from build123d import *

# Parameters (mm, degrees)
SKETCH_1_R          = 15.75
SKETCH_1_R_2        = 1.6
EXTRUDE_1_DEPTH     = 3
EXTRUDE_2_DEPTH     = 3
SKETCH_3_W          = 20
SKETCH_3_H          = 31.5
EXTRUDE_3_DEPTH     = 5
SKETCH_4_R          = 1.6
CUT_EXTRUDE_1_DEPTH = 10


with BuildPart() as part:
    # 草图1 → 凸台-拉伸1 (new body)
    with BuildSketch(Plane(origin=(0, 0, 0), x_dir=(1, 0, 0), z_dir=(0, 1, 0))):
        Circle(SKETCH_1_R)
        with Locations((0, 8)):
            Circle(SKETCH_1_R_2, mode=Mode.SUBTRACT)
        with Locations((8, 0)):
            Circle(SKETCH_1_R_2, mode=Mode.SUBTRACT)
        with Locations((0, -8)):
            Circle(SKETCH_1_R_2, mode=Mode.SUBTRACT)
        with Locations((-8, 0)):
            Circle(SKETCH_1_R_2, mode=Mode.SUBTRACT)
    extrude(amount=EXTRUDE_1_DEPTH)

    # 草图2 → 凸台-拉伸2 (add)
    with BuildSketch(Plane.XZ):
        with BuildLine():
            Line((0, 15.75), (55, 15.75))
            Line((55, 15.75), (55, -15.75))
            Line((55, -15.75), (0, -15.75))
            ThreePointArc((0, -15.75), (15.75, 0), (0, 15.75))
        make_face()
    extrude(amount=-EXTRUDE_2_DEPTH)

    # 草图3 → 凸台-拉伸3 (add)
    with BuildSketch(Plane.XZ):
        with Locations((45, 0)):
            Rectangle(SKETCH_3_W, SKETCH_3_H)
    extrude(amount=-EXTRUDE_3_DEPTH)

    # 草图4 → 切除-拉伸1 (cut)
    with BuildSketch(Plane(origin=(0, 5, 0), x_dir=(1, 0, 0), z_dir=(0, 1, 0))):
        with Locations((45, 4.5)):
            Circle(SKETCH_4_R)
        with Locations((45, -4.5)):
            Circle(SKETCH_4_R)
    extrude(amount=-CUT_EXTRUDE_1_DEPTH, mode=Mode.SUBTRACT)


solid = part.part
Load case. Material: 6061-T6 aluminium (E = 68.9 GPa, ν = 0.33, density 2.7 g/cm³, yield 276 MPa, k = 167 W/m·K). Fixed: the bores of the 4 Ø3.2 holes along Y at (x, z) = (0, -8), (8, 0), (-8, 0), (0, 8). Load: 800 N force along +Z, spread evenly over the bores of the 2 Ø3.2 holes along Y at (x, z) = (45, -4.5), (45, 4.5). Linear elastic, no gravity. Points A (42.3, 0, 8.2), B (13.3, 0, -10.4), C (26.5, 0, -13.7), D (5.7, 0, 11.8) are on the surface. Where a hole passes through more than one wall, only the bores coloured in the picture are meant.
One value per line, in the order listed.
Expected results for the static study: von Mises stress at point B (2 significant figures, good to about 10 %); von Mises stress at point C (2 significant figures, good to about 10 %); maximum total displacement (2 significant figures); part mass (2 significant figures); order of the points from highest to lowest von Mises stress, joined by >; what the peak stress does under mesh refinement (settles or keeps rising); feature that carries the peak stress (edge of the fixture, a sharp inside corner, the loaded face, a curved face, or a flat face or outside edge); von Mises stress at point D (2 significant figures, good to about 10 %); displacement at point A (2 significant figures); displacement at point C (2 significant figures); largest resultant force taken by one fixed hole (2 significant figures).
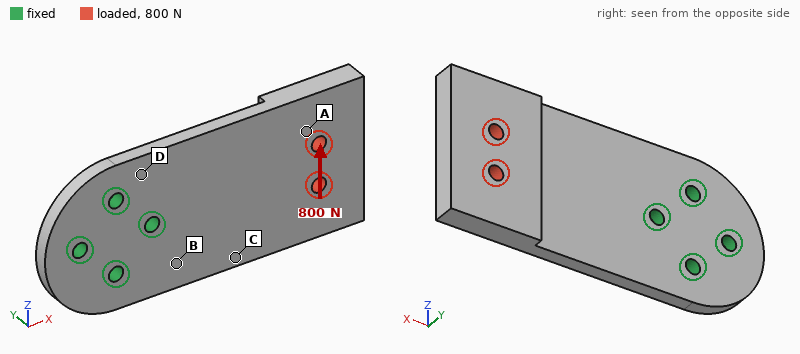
38 MPa
21 MPa
97 µm
20 g
D > B > C > A
keeps rising
edge of the fixture
53 MPa
59 µm
42 µm
1.3 kN
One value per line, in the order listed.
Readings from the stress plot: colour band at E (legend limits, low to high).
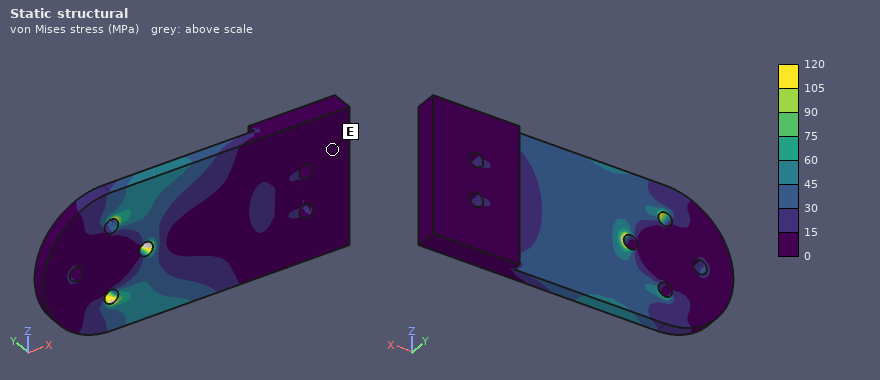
0 to 15 MPa
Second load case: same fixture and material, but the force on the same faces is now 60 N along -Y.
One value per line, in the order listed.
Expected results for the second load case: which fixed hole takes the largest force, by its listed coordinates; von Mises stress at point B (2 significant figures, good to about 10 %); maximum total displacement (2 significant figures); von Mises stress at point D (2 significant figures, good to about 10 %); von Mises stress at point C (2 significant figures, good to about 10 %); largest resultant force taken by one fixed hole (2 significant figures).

(8, 0)
34 MPa
0.29 mm
17 MPa
24 MPa
190 N
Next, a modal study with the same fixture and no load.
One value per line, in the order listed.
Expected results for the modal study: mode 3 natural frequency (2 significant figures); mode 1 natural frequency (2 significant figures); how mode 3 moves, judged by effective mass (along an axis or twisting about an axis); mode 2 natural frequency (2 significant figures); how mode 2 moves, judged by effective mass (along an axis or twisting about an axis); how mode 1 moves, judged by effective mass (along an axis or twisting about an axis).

5600 Hz
880 Hz
along Z
2800 Hz
twisting about X
along Y
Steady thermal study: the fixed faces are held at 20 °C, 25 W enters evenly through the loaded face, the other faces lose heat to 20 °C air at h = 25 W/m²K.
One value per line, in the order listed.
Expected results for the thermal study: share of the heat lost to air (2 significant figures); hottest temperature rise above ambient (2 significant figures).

13 %
56 K
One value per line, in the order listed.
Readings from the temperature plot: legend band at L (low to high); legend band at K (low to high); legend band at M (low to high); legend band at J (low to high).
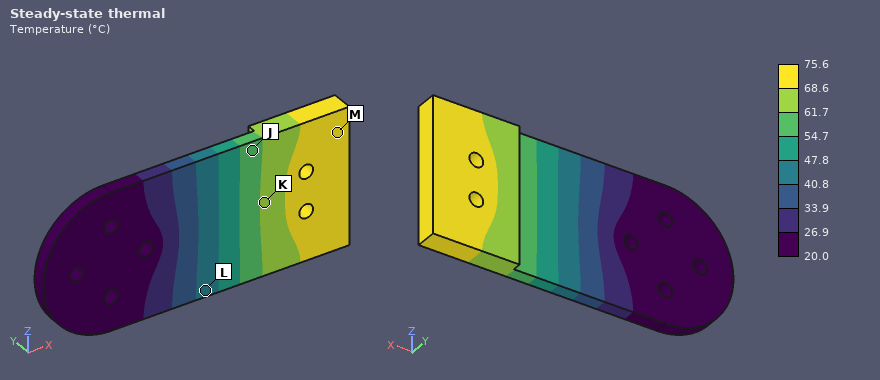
40.8 to 47.8 °C
61.7 to 68.6 °C
68.6 to 75.6 °C
54.7 to 61.7 °C
